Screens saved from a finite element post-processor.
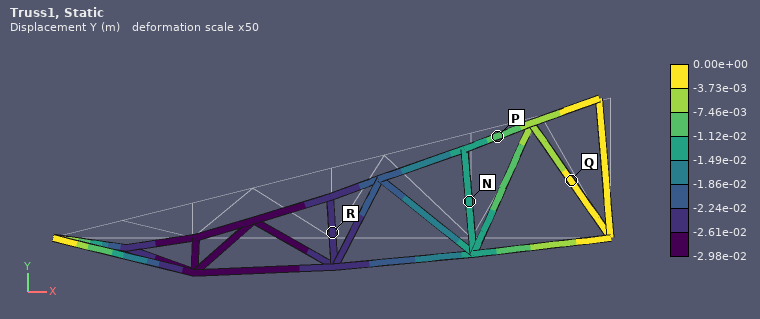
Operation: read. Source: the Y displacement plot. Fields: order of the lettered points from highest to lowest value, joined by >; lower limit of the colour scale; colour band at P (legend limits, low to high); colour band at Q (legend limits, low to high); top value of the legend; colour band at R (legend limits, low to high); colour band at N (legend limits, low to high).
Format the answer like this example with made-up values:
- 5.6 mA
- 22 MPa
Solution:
- Q > P > N > R
- -2.98e-02 m
- -1.12e-02 to -7.46e-03 m
- -3.73e-03 to 0.00e+00 m
- 0.00e+00 m
- -2.61e-02 to -2.24e-02 m
- -1.49e-02 to -1.12e-02 m
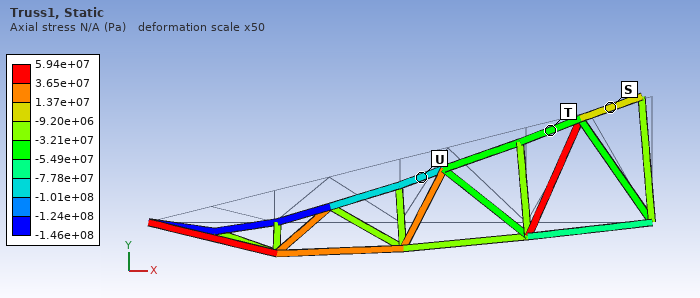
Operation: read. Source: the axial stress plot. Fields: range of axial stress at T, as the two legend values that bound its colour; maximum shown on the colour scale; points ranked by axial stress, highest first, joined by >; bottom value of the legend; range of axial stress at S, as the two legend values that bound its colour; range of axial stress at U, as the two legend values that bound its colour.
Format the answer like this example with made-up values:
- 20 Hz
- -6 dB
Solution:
- -5.49e+07 to -3.21e+07 Pa
- 5.94e+07 Pa
- S > T > U
- -1.46e+08 Pa
- -9.20e+06 to 1.37e+07 Pa
- -1.01e+08 to -7.78e+07 Pa
